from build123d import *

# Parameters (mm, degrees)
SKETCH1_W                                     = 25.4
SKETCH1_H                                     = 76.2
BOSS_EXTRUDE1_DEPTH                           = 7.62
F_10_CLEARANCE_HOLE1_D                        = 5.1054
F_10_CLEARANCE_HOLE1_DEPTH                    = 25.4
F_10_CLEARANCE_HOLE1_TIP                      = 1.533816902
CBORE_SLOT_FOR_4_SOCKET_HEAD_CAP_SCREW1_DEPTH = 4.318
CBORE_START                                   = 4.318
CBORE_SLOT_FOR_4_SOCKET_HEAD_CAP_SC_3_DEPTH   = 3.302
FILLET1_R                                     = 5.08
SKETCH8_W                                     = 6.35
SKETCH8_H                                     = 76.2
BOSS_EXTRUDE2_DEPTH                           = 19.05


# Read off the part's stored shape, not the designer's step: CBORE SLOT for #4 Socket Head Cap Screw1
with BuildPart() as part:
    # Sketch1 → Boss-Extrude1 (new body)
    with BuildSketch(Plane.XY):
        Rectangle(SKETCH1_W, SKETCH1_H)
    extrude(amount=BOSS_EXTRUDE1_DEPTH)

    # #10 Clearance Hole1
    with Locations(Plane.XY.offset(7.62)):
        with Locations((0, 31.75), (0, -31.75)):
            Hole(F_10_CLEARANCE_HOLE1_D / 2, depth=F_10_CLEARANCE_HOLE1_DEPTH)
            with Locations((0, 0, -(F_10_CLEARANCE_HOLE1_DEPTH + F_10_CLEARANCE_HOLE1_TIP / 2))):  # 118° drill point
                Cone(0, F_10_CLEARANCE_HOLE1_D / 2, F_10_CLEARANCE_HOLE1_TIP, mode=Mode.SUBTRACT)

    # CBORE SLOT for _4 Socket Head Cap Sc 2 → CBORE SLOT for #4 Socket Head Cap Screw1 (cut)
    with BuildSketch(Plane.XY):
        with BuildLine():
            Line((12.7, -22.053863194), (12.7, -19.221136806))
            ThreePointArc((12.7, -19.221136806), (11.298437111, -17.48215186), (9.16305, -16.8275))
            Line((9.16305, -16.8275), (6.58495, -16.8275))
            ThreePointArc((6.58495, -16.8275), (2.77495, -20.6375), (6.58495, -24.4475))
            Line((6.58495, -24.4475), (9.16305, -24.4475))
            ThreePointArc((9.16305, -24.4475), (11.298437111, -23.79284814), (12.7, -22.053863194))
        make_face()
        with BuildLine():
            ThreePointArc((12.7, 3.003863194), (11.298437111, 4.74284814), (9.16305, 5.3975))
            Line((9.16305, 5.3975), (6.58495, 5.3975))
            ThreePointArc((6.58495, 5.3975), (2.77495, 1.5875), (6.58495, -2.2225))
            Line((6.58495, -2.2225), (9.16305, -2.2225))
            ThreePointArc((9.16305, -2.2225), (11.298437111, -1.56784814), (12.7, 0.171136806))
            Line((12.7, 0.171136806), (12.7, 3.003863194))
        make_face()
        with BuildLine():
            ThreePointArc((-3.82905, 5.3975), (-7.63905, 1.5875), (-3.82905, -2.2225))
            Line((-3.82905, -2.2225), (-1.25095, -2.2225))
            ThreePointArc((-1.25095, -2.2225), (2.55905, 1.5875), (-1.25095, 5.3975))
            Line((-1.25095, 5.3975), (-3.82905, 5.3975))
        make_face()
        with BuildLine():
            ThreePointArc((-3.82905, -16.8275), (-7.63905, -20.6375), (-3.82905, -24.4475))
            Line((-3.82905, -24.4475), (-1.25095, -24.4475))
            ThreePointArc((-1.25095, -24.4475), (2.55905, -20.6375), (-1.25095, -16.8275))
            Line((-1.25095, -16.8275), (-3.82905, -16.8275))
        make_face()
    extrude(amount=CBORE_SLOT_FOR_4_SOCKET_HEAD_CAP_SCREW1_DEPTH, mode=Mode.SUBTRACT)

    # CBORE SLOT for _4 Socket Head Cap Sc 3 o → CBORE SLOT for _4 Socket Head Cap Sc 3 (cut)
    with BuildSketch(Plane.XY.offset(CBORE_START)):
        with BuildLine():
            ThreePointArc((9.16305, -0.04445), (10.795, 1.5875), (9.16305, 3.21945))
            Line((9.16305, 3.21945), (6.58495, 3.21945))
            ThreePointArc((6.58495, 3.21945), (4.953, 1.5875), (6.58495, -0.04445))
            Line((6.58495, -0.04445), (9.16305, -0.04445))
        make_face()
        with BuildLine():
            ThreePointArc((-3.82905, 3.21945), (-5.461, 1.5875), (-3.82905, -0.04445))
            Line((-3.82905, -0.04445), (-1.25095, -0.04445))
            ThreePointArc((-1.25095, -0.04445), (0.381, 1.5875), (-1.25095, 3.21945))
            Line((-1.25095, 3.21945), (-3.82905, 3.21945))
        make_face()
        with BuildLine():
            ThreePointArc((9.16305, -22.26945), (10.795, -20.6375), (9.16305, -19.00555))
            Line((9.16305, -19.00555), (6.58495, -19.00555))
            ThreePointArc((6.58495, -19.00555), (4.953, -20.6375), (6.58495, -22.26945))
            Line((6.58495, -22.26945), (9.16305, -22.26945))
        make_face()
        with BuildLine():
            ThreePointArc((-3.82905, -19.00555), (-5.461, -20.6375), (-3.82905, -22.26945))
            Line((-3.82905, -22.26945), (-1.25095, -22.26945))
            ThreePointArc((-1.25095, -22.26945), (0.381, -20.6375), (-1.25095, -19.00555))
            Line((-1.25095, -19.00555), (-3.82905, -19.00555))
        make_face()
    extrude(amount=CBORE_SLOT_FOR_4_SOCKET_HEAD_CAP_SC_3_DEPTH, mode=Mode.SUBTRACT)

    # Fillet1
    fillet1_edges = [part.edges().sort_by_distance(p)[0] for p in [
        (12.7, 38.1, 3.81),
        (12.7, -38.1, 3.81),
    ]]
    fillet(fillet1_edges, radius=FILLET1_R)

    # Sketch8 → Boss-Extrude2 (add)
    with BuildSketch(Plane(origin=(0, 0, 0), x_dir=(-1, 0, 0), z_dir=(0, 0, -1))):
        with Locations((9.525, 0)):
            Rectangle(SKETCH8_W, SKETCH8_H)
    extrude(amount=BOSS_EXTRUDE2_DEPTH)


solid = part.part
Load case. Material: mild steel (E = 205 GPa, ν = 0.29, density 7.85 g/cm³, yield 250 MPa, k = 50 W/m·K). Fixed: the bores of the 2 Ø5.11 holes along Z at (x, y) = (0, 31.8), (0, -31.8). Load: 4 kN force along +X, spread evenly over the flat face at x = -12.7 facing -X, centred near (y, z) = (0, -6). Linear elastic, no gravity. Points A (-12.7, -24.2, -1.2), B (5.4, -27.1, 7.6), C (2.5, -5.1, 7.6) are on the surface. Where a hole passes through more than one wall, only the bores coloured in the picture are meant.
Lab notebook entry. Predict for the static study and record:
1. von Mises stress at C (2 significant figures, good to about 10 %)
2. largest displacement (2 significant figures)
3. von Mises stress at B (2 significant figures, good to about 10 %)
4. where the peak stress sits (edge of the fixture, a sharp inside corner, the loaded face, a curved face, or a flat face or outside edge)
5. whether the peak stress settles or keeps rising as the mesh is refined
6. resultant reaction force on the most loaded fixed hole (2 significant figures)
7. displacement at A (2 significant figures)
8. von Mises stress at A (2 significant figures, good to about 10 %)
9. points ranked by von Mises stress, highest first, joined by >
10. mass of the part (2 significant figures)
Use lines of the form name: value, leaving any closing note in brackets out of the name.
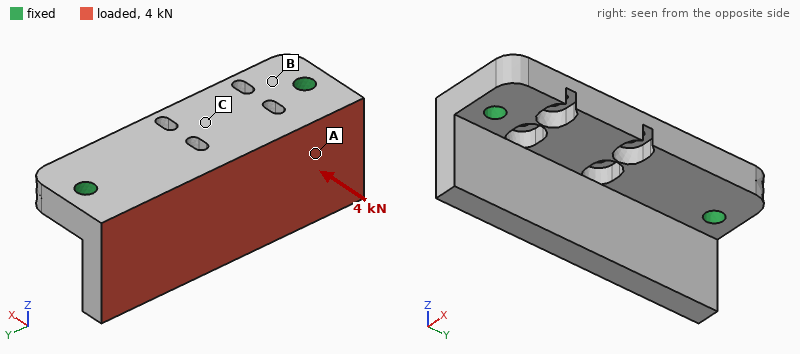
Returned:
von Mises stress at C: 15 MPa
largest displacement: 50 µm
von Mises stress at B: 26 MPa
where the peak stress sits: edge of the fixture
whether the peak stress settles or keeps rising as the mesh is refined: keeps rising
resultant reaction force on the most loaded fixed hole: 2.1 kN
displacement at A: 15 µm
von Mises stress at A: 50 MPa
points ranked by von Mises stress, highest first, joined by >: A > B > C
mass of the part: 170 g
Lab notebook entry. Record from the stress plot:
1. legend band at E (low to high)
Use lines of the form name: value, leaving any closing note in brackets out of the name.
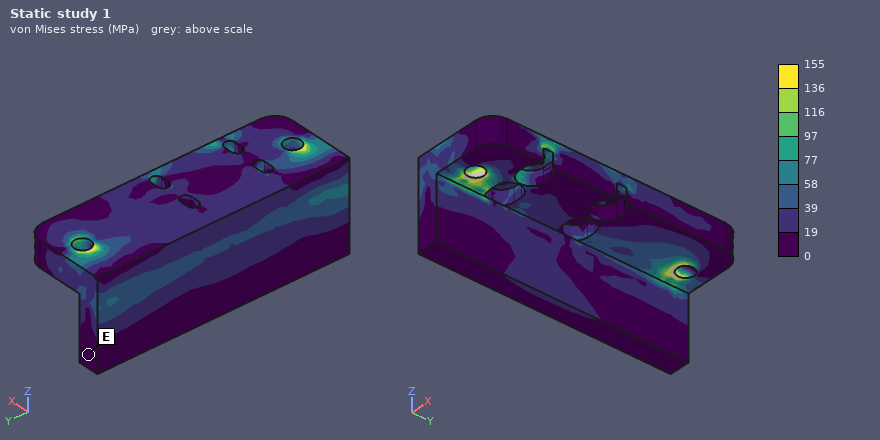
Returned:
legend band at E: 0 to 19 MPa
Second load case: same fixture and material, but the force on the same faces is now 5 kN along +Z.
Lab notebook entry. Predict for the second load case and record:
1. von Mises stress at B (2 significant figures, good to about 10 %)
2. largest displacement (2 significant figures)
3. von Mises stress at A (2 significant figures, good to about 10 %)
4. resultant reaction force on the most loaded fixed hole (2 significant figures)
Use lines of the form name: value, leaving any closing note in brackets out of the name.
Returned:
von Mises stress at B: 30 MPa
largest displacement: 45 µm
von Mises stress at A: 38 MPa
resultant reaction force on the most loaded fixed hole: 2.6 kN
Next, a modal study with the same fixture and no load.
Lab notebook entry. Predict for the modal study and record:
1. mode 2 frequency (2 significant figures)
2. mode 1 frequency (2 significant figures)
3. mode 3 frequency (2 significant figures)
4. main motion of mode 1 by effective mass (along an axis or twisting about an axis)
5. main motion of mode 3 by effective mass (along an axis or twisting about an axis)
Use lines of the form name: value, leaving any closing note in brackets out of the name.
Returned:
mode 2 frequency: 9200 Hz
mode 1 frequency: 5400 Hz
mode 3 frequency: 9800 Hz
main motion of mode 1 by effective mass: along X
main motion of mode 3 by effective mass: along Z
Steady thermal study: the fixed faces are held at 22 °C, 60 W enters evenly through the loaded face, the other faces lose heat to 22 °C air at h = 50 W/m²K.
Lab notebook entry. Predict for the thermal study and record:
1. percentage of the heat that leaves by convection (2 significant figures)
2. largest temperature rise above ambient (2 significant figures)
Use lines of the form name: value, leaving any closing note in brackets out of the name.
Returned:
percentage of the heat that leaves by convection: 18 %
largest temperature rise above ambient: 59 K
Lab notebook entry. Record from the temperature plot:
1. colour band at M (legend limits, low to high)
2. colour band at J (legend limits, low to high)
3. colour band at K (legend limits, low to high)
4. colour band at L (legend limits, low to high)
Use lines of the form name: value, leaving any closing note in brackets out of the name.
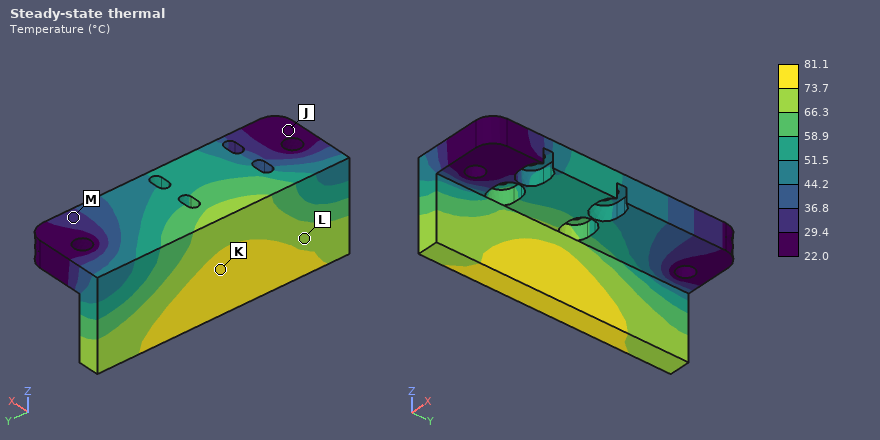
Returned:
colour band at M: 29.4 to 36.8 °C
colour band at J: 22.0 to 29.4 °C
colour band at K: 73.7 to 81.1 °C
colour band at L: 66.3 to 73.7 °C
